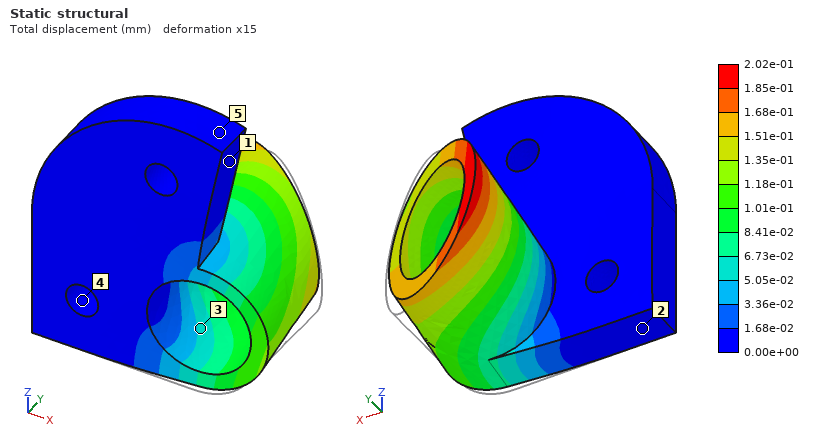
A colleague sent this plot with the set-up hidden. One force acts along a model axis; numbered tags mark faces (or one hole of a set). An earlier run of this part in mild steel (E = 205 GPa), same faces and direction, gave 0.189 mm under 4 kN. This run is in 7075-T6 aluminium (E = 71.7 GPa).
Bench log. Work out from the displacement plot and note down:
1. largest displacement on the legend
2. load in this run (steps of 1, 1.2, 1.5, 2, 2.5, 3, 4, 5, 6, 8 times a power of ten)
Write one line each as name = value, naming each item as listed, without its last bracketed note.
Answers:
largest displacement on the legend = 2.02e-01 mm
load in this run = 1.5 kN
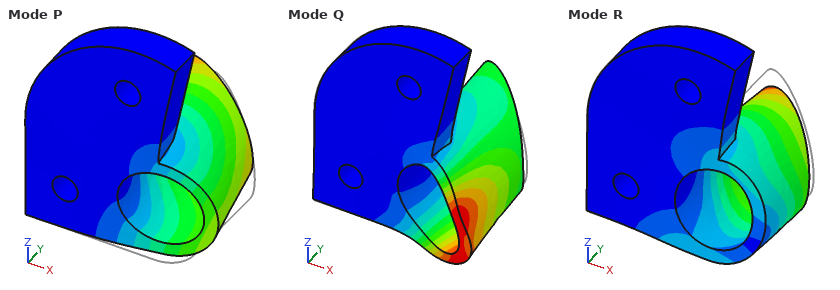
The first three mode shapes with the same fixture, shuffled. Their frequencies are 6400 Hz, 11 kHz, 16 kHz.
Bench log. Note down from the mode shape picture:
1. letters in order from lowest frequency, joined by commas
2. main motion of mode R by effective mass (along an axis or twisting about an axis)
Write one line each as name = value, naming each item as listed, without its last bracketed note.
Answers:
letters in order from lowest frequency, joined by commas = P, R, Q
main motion of mode R by effective mass = along Z
